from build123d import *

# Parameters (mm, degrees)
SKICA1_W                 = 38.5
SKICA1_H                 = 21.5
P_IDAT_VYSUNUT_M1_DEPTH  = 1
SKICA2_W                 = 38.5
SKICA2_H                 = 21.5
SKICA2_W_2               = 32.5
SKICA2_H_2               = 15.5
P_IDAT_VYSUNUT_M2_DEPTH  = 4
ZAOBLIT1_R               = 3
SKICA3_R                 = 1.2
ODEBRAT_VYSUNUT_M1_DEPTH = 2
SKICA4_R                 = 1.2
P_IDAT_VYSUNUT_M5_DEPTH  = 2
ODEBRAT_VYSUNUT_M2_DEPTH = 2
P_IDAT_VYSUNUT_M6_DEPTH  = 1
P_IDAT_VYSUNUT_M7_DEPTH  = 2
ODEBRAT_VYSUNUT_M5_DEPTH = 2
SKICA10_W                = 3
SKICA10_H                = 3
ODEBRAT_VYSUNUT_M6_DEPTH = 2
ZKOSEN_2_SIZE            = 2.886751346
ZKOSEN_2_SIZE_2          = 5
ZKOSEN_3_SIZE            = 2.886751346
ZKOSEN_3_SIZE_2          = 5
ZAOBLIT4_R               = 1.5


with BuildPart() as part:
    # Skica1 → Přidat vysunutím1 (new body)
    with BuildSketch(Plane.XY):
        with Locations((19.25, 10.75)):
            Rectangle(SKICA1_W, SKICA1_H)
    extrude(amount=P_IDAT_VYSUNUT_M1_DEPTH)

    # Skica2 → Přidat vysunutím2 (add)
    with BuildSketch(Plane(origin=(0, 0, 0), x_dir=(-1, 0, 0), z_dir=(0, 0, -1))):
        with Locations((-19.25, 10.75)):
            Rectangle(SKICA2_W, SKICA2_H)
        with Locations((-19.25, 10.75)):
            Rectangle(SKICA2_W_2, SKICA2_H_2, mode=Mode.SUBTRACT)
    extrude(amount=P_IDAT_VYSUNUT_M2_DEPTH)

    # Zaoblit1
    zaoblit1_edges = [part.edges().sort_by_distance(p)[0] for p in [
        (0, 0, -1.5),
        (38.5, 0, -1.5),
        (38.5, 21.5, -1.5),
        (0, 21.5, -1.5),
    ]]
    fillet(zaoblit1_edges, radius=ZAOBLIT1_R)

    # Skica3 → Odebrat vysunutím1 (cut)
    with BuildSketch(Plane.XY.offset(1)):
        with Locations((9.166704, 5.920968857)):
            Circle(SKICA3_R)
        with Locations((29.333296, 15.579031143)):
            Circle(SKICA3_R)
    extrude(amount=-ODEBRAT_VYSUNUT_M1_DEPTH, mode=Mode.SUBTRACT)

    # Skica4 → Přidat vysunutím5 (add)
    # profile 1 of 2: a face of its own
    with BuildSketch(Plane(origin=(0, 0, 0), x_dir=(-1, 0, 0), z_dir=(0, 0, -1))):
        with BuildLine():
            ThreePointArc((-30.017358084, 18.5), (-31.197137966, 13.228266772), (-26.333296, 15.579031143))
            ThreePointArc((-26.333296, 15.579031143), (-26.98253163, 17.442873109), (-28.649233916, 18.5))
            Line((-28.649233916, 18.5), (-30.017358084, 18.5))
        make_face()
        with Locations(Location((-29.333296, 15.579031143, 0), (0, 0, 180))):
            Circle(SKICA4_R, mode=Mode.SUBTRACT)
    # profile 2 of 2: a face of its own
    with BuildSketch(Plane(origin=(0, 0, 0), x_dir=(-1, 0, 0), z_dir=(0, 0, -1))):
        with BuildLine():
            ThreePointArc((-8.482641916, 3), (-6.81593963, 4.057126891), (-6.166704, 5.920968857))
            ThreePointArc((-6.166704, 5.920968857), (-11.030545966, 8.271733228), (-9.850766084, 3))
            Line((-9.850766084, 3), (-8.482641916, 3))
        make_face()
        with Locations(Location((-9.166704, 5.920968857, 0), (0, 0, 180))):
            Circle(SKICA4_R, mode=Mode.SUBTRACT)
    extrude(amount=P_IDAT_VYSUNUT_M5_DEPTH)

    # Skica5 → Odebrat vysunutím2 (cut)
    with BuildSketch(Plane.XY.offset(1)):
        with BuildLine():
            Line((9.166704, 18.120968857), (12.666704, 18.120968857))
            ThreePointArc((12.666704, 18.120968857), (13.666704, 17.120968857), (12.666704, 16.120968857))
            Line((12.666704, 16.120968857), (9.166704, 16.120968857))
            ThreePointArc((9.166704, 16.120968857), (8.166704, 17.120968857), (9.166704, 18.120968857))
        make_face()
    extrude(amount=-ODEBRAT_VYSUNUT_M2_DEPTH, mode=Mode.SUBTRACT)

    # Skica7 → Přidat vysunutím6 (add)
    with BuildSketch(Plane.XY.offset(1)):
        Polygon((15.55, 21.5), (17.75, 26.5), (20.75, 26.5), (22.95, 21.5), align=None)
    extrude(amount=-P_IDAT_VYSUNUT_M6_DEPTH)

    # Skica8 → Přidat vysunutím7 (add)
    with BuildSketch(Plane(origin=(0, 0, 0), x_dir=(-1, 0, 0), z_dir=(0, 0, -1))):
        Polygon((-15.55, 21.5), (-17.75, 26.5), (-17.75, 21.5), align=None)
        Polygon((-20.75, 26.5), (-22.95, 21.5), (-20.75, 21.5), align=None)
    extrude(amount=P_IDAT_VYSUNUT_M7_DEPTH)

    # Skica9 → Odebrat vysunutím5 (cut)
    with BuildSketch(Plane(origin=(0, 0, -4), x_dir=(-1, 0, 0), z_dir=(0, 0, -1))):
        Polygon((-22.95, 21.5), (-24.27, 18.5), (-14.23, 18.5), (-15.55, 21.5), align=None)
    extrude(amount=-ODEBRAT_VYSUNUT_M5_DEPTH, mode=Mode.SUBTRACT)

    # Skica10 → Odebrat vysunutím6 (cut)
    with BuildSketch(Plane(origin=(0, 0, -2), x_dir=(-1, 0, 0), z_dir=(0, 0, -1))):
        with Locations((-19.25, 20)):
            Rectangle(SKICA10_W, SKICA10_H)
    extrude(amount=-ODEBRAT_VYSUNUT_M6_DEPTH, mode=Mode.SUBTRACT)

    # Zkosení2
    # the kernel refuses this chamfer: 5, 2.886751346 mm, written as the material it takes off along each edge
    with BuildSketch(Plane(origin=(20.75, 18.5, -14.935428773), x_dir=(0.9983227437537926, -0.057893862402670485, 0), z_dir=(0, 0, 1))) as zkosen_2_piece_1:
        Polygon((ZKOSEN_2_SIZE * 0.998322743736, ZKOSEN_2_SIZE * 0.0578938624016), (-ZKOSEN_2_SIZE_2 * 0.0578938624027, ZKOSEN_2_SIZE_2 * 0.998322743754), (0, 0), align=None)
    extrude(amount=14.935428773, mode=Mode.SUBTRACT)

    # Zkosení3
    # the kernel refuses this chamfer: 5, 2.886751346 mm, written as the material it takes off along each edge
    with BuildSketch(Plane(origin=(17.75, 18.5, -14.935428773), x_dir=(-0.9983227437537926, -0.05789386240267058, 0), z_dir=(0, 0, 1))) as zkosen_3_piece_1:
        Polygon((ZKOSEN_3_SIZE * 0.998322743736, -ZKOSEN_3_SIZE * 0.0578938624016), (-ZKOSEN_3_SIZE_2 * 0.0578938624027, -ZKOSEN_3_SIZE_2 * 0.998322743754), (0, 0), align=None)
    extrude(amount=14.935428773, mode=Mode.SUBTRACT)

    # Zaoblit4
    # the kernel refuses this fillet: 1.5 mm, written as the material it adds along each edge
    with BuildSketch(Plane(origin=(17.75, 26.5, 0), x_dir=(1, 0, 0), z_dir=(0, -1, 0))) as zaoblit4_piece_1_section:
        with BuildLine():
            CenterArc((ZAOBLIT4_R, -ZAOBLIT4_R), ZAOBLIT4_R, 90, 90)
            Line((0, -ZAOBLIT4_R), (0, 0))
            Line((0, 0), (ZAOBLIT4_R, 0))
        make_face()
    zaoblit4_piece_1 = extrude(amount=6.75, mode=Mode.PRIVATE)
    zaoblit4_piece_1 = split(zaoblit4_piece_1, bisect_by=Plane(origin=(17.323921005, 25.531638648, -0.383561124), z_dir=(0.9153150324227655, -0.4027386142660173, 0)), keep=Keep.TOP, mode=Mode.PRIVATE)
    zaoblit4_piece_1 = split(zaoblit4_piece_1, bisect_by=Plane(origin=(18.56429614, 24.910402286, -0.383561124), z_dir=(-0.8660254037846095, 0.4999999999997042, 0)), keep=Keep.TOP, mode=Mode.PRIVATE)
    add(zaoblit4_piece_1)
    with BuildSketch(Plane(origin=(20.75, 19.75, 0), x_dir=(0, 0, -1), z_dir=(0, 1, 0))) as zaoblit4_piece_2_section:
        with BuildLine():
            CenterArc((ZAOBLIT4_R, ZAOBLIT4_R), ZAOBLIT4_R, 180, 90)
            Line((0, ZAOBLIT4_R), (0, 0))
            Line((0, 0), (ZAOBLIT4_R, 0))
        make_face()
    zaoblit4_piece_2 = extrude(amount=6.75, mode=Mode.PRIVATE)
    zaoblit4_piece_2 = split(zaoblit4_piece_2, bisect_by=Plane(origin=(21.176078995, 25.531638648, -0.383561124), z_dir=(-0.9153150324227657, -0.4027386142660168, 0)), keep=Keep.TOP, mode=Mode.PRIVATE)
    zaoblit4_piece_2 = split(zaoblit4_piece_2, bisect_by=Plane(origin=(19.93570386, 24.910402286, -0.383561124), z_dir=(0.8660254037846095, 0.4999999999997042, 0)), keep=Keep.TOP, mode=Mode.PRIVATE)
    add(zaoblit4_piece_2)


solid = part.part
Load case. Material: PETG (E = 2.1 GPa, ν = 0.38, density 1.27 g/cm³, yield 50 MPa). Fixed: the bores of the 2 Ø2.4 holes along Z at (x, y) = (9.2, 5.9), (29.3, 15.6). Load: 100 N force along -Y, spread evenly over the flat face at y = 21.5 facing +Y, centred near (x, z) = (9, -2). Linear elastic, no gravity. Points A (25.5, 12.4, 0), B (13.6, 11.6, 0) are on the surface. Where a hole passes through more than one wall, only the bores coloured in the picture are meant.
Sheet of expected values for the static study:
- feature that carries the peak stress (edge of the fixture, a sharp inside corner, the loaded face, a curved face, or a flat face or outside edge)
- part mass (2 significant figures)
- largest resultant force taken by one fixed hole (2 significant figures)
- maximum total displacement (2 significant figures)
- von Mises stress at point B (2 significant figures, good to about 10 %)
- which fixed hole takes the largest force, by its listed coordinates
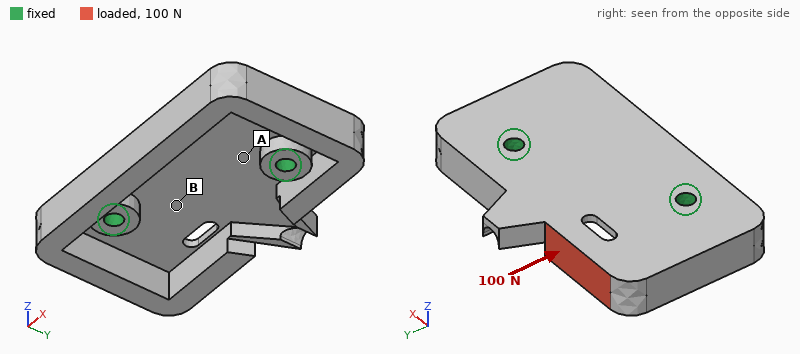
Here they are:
a curved face
2.7 g
94 N
0.53 mm
7.1 MPa
(9.2, 5.9)
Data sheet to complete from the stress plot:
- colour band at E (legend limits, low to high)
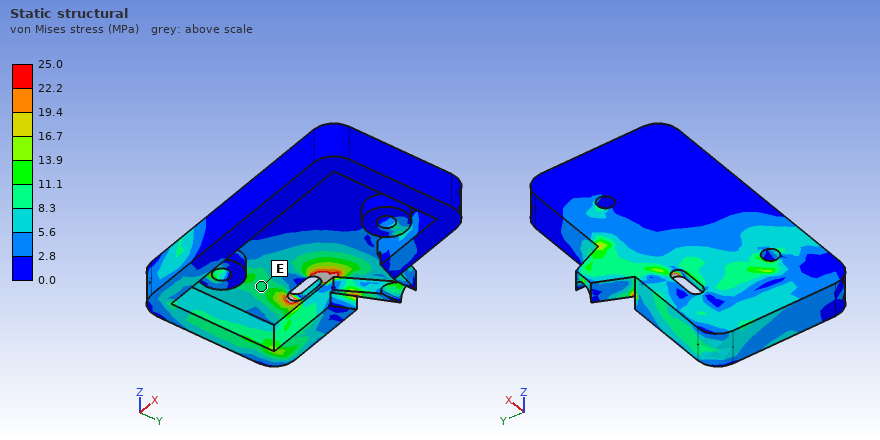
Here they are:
8.3 to 11.1 MPa
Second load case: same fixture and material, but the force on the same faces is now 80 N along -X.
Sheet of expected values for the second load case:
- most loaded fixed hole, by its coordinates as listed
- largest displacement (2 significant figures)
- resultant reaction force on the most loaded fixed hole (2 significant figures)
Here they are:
(29.3, 15.6)
0.53 mm
67 N
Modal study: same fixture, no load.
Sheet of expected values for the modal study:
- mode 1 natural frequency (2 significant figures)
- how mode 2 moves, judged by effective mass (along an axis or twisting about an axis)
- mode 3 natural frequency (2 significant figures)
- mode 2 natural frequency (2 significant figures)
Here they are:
1300 Hz
along Z
2800 Hz
1700 Hz
